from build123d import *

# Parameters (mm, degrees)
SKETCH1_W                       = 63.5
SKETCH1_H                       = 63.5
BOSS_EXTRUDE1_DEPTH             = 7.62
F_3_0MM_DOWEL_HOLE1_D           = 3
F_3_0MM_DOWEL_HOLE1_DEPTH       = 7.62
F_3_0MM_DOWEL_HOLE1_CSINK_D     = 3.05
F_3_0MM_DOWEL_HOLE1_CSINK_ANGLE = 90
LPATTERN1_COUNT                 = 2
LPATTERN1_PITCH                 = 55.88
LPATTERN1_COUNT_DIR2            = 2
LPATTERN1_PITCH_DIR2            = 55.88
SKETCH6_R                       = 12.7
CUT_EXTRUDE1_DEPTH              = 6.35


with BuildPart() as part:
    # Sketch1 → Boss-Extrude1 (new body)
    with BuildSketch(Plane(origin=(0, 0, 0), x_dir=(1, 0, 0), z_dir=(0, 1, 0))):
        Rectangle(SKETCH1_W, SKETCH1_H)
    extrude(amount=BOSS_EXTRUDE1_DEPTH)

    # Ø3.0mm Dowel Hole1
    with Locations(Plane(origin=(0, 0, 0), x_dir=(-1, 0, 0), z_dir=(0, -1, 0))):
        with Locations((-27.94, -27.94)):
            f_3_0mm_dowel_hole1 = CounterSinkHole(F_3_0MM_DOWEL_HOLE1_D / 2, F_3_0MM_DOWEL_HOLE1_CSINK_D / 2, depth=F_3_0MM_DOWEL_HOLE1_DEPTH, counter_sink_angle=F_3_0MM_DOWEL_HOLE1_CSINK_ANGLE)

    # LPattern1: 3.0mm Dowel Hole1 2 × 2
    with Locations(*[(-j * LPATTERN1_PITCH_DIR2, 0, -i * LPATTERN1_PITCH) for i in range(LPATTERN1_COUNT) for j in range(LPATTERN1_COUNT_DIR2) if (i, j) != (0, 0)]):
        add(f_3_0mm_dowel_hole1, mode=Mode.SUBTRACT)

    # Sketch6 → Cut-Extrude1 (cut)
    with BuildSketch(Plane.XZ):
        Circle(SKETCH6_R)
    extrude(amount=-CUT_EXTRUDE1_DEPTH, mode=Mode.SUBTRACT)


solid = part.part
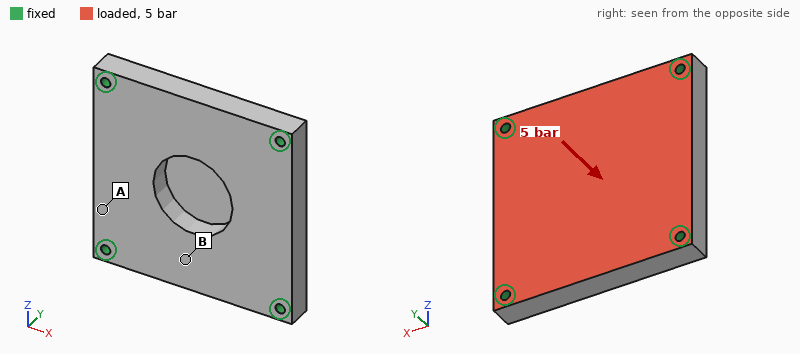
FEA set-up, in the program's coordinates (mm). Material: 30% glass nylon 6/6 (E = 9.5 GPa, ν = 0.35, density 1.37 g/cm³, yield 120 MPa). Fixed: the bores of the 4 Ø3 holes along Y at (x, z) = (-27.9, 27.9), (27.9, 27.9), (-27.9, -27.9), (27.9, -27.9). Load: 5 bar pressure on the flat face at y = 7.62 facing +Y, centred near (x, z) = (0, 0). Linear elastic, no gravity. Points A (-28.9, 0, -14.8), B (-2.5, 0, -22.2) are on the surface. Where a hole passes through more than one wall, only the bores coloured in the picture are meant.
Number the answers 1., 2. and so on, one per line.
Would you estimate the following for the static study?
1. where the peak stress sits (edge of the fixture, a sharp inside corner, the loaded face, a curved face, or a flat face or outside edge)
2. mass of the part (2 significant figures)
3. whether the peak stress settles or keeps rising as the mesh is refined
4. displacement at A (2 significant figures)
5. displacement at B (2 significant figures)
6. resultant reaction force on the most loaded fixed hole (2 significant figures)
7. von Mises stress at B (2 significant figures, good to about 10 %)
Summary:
1. edge of the fixture
2. 37 g
3. keeps rising
4. 0.051 mm
5. 0.11 mm
6. 510 N
7. 12 MPa
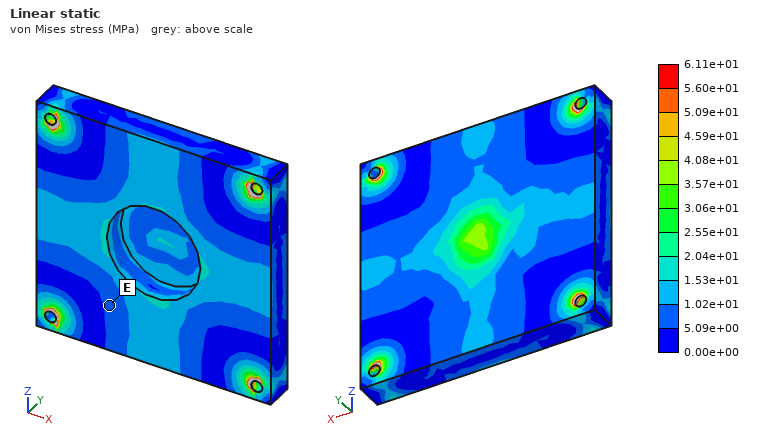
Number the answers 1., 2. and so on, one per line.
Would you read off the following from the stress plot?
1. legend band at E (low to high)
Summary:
1. 5.09e+00 to 1.02e+01 MPa
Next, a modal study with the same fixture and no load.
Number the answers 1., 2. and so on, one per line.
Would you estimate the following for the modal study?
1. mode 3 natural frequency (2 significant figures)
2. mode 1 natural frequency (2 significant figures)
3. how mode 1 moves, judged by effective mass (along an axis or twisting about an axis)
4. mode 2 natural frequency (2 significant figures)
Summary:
1. 5900 Hz
2. 3800 Hz
3. along Y
4. 5900 Hz
